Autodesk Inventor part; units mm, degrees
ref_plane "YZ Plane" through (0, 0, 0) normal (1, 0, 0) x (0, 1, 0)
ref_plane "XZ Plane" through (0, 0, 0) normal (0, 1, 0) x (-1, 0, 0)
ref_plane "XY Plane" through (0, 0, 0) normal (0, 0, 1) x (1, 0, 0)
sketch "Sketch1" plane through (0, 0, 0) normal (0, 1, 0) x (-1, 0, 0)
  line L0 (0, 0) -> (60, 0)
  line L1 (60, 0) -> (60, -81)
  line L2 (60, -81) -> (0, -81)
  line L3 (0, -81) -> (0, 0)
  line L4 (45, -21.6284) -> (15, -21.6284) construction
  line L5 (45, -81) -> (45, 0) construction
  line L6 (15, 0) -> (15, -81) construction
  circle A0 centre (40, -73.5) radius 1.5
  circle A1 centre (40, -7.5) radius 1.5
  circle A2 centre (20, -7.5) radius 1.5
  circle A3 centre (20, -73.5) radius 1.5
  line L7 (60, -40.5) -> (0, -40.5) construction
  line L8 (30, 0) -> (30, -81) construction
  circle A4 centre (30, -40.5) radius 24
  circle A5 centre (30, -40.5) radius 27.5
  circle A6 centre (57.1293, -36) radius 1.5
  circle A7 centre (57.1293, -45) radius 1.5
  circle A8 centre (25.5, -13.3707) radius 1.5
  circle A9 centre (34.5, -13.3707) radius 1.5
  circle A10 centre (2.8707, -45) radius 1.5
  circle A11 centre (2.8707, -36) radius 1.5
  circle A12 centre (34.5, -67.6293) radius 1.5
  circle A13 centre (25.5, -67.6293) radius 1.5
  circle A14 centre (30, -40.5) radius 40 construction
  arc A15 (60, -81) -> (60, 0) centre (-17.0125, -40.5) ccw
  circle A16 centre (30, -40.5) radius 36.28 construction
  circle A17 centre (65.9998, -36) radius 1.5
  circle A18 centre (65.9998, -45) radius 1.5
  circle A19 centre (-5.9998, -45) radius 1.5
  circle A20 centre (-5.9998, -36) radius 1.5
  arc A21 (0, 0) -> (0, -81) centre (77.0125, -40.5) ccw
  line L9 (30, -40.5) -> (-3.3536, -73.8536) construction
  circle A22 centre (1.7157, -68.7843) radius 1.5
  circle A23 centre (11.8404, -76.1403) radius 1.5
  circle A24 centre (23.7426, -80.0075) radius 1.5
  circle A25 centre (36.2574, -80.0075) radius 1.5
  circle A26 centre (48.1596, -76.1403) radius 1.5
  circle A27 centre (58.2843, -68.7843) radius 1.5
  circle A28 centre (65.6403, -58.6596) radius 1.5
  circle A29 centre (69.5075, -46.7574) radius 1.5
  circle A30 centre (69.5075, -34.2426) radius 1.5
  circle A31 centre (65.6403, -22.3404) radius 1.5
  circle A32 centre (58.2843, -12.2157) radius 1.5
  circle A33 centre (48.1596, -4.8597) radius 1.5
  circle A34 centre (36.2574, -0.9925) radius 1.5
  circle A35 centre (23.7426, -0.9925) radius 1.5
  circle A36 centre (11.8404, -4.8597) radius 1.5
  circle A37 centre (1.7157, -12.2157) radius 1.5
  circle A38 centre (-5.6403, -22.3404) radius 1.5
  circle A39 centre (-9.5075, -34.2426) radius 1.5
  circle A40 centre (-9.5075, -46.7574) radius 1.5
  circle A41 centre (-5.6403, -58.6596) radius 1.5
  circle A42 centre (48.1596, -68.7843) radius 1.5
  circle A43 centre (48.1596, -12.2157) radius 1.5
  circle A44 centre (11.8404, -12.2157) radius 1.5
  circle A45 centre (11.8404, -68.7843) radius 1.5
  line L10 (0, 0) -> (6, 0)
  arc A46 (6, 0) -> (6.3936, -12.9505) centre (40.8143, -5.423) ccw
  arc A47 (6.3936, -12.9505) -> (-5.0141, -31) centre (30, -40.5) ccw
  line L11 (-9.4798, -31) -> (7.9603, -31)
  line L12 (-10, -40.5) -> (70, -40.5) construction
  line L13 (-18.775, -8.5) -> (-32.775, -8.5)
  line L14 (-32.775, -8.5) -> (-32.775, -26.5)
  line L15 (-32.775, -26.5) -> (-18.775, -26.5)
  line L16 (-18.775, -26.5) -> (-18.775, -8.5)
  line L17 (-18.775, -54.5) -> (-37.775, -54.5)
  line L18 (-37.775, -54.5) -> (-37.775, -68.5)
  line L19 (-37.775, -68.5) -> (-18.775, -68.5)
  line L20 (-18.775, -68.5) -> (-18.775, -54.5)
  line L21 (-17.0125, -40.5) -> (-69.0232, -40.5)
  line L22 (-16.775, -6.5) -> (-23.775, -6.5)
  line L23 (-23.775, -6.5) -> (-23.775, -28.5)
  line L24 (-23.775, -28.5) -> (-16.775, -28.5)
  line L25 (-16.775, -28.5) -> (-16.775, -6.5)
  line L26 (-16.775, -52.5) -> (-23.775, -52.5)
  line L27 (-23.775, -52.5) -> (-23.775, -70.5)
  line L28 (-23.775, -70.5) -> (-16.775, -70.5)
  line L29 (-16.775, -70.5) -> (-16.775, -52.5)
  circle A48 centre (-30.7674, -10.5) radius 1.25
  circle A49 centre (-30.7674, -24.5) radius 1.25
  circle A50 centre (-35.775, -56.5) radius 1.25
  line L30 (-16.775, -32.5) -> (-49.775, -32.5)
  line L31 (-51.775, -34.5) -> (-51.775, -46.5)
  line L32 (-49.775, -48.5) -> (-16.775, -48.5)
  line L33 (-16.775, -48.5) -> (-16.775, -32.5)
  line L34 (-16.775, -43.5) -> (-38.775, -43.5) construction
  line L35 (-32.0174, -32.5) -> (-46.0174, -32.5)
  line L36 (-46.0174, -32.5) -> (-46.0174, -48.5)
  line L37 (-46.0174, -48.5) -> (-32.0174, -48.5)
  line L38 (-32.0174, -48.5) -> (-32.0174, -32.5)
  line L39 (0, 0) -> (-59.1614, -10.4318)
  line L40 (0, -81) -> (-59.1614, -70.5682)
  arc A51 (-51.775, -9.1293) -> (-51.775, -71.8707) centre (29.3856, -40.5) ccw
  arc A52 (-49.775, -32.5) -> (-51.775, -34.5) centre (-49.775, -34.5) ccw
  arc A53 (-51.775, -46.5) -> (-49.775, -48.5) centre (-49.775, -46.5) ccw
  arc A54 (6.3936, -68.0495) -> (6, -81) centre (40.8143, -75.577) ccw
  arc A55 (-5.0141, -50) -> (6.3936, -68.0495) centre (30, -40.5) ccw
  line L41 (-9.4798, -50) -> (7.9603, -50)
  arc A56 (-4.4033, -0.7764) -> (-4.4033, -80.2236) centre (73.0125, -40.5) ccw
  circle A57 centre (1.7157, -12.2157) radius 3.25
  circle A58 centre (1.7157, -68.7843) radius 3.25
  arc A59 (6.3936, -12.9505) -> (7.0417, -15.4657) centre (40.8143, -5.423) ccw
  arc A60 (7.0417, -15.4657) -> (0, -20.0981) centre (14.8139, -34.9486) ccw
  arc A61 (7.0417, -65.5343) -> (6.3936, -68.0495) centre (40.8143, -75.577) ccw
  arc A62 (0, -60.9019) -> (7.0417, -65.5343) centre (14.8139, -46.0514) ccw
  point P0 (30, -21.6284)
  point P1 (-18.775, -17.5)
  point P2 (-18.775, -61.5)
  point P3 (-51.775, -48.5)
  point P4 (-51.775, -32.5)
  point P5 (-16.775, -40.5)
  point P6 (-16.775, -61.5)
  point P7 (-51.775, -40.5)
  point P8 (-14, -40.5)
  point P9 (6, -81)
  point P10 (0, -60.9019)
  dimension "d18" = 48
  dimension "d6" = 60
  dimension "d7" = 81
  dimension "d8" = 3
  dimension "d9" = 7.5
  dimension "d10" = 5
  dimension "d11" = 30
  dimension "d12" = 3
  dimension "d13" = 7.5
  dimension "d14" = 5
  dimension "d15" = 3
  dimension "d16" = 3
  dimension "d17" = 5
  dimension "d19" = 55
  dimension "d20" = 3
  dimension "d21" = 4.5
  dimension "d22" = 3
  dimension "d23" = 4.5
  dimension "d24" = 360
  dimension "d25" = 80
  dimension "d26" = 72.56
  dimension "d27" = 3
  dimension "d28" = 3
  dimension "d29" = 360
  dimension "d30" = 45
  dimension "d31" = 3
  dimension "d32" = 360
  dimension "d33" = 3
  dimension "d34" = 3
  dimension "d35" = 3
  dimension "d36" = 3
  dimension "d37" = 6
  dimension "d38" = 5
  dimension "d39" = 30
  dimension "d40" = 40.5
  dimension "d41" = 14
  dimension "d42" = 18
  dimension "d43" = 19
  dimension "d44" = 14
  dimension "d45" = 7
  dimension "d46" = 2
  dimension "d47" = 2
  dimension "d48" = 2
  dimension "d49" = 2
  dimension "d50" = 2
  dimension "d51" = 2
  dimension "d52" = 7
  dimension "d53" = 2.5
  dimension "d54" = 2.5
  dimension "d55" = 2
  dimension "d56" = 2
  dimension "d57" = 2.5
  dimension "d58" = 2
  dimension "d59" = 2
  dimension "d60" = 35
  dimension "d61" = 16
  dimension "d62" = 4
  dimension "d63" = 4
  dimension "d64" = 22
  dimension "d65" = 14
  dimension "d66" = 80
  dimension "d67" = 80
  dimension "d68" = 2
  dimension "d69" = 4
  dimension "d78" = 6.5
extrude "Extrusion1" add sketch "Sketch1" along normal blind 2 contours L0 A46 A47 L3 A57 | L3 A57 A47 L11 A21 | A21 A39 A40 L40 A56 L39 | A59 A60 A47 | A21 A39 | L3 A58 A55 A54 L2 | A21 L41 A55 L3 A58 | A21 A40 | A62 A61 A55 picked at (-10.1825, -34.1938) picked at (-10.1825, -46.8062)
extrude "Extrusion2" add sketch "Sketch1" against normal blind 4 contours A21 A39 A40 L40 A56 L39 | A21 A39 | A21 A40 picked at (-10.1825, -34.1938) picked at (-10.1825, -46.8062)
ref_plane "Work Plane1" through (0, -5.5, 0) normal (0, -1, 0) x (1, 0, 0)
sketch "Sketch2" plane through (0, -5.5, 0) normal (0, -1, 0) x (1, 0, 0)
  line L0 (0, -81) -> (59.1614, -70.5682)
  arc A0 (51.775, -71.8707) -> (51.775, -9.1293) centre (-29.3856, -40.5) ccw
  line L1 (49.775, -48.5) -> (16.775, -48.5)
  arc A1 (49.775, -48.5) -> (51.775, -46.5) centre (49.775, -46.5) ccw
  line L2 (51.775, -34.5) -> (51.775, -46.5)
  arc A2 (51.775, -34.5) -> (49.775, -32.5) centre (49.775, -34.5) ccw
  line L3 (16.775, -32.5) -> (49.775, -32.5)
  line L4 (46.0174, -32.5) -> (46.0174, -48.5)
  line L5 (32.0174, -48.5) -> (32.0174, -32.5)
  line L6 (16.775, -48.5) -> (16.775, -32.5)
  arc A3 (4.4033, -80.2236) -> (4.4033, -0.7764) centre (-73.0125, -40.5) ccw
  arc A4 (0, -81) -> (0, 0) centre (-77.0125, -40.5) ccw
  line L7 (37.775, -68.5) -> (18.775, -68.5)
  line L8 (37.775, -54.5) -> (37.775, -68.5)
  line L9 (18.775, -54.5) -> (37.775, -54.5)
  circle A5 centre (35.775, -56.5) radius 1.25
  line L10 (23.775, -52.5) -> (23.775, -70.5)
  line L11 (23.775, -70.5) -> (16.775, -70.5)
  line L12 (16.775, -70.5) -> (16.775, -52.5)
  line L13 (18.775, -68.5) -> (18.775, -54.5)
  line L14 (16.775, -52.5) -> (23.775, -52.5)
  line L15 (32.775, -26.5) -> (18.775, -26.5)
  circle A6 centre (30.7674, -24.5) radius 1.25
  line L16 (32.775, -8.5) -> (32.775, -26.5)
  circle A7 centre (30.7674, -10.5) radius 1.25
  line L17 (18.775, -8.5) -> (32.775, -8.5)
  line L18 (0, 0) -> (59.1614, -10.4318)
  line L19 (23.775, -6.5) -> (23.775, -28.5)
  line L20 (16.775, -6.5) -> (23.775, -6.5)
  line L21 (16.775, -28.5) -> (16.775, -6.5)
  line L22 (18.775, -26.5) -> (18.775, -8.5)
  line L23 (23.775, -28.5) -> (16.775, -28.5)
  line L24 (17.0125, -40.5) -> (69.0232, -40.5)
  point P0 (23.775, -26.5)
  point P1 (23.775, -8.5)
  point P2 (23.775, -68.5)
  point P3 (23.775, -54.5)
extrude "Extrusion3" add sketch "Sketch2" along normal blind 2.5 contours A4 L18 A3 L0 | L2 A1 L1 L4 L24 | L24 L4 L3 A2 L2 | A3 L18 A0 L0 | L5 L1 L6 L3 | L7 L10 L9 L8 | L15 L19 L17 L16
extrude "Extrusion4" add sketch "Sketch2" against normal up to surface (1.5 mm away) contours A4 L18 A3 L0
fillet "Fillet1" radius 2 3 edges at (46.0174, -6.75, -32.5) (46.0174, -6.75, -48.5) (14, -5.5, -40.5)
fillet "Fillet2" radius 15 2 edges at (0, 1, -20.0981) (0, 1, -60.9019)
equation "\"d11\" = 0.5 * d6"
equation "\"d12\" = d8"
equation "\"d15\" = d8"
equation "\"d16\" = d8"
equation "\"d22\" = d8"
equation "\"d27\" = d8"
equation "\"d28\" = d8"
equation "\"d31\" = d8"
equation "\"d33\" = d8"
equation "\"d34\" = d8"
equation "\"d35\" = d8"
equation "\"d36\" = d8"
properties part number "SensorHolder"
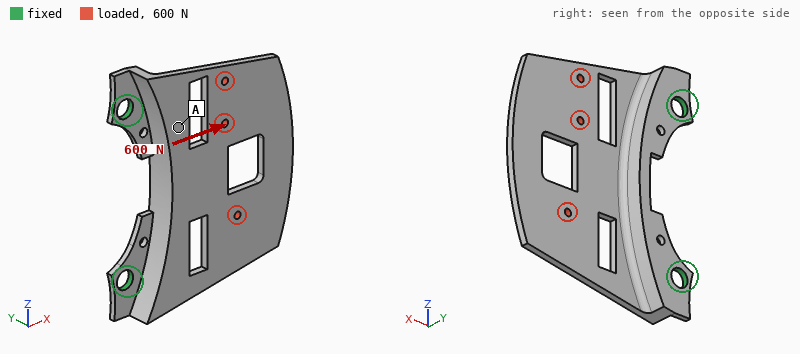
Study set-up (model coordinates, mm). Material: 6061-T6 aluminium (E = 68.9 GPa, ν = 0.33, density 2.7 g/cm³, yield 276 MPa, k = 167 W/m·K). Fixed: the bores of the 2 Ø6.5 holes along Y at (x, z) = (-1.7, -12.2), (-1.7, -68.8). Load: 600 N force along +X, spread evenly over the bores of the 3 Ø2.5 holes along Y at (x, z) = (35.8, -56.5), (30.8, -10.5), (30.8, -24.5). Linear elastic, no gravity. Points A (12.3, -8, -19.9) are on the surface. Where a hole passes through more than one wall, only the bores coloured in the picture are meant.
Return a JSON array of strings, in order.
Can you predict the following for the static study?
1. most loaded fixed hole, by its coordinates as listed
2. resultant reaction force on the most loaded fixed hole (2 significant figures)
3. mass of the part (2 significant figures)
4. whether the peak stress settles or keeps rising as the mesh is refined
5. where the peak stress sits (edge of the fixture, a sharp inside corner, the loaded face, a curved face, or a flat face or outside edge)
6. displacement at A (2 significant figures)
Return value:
["(-1.7, -12.2)", "410 N", "29 g", "keeps rising", "edge of the fixture", "0.15 mm"]
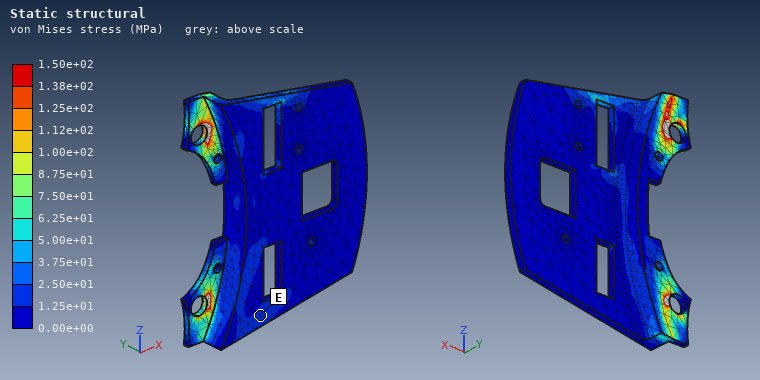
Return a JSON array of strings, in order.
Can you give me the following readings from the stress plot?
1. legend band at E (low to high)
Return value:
["1.25e+01 to 2.50e+01 MPa"]
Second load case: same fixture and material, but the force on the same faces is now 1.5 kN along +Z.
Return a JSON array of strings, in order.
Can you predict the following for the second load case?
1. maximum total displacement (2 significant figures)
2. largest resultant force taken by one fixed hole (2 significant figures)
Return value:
["0.18 mm", "1.1 kN"]
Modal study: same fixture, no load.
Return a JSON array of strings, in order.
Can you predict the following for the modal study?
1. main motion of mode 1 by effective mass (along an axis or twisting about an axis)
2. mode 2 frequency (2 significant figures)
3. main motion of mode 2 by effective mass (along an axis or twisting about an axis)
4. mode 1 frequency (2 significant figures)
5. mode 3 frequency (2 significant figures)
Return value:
["along Y", "1500 Hz", "twisting about X", "550 Hz", "2600 Hz"]
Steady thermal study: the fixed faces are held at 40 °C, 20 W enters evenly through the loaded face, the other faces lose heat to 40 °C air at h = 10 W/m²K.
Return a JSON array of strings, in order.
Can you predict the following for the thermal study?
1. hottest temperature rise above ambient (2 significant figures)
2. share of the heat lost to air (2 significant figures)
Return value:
["57 K", "13 %"]
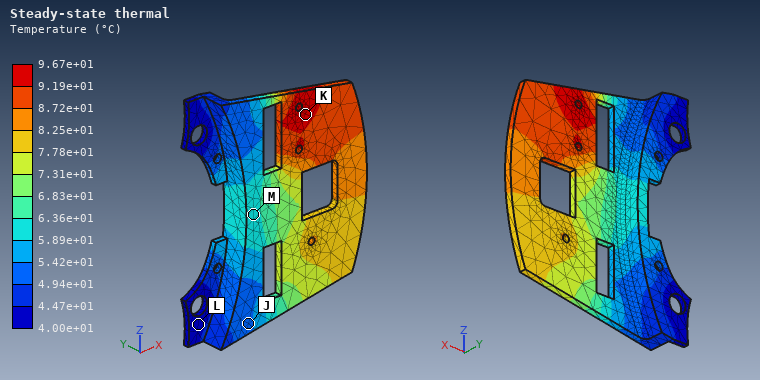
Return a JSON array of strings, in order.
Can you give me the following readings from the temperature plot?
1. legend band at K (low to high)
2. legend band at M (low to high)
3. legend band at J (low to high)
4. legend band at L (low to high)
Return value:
["9.19e+01 to 9.67e+01 °C", "5.89e+01 to 6.36e+01 °C", "4.94e+01 to 5.42e+01 °C", "4.00e+01 to 4.47e+01 °C"]
